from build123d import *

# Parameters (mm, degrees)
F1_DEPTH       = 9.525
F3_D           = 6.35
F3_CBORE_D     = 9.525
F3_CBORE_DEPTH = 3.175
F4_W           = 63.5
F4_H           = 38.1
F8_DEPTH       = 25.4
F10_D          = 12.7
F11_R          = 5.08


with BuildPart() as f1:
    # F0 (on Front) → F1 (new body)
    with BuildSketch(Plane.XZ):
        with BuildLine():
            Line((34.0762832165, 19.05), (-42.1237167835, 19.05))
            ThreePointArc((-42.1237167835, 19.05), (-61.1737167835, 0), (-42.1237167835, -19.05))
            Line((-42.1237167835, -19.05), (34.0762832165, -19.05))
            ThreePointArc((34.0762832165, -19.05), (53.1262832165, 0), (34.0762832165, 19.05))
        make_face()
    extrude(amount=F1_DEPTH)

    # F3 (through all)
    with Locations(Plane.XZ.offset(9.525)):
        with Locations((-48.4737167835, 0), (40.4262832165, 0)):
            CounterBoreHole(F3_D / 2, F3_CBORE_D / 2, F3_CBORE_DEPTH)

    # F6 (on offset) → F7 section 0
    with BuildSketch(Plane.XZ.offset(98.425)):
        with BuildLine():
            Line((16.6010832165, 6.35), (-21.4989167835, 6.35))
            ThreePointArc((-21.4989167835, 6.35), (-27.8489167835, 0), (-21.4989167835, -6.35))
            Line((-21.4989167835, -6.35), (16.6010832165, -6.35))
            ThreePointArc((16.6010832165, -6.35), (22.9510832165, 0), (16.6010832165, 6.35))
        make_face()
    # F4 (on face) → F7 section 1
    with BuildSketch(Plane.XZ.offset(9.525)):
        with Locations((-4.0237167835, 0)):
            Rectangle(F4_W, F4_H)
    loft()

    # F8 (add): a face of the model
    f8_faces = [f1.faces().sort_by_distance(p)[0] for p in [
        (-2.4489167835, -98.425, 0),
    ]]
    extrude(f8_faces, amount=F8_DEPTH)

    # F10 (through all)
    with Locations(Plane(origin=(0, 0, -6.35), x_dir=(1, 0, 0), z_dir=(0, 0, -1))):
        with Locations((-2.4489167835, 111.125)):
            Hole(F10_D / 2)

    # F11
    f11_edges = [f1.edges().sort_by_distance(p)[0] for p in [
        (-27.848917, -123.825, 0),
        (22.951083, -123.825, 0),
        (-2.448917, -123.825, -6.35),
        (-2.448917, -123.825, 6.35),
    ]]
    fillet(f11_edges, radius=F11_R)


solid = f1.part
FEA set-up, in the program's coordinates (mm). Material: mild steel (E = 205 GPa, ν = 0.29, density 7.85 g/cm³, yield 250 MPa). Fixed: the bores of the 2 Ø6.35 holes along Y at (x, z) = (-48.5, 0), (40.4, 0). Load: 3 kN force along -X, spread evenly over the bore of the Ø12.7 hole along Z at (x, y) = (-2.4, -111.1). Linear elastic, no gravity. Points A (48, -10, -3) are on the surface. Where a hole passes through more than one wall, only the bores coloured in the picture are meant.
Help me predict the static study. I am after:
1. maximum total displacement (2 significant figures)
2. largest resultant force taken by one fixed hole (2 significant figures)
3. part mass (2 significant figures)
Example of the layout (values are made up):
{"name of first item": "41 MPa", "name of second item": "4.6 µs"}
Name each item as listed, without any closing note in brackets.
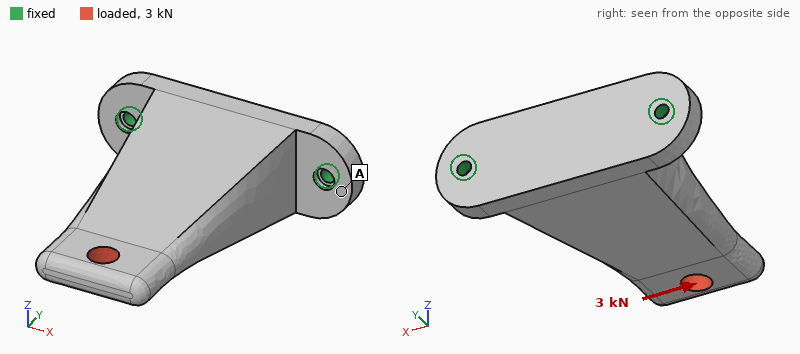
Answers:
{"maximum total displacement": "50 µm", "largest resultant force taken by one fixed hole": "4.3 kN", "part mass": "1.4 kg"}
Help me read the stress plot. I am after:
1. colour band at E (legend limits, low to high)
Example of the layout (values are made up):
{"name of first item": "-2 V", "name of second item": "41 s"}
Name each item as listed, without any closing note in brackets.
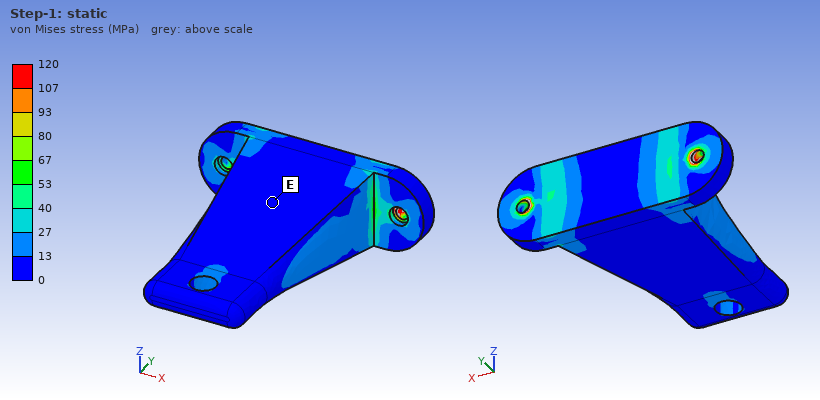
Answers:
{"colour band at E": "0 to 13 MPa"}
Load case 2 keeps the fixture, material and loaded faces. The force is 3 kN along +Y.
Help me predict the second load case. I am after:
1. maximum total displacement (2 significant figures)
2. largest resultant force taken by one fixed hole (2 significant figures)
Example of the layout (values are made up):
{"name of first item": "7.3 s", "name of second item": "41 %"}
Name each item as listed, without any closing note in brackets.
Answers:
{"maximum total displacement": "6.4 µm", "largest resultant force taken by one fixed hole": "1.9 kN"}
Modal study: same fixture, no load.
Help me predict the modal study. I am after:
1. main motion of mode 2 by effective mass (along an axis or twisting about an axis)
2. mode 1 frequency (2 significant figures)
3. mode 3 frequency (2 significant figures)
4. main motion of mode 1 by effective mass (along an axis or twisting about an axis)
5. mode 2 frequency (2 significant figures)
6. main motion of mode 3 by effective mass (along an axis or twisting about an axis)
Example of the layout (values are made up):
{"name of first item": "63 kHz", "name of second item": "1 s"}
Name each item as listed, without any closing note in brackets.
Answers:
{"main motion of mode 2 by effective mass": "along X", "mode 1 frequency": "650 Hz", "mode 3 frequency": "3800 Hz", "main motion of mode 1 by effective mass": "along Z", "mode 2 frequency": "2600 Hz", "main motion of mode 3 by effective mass": "along Y"}
